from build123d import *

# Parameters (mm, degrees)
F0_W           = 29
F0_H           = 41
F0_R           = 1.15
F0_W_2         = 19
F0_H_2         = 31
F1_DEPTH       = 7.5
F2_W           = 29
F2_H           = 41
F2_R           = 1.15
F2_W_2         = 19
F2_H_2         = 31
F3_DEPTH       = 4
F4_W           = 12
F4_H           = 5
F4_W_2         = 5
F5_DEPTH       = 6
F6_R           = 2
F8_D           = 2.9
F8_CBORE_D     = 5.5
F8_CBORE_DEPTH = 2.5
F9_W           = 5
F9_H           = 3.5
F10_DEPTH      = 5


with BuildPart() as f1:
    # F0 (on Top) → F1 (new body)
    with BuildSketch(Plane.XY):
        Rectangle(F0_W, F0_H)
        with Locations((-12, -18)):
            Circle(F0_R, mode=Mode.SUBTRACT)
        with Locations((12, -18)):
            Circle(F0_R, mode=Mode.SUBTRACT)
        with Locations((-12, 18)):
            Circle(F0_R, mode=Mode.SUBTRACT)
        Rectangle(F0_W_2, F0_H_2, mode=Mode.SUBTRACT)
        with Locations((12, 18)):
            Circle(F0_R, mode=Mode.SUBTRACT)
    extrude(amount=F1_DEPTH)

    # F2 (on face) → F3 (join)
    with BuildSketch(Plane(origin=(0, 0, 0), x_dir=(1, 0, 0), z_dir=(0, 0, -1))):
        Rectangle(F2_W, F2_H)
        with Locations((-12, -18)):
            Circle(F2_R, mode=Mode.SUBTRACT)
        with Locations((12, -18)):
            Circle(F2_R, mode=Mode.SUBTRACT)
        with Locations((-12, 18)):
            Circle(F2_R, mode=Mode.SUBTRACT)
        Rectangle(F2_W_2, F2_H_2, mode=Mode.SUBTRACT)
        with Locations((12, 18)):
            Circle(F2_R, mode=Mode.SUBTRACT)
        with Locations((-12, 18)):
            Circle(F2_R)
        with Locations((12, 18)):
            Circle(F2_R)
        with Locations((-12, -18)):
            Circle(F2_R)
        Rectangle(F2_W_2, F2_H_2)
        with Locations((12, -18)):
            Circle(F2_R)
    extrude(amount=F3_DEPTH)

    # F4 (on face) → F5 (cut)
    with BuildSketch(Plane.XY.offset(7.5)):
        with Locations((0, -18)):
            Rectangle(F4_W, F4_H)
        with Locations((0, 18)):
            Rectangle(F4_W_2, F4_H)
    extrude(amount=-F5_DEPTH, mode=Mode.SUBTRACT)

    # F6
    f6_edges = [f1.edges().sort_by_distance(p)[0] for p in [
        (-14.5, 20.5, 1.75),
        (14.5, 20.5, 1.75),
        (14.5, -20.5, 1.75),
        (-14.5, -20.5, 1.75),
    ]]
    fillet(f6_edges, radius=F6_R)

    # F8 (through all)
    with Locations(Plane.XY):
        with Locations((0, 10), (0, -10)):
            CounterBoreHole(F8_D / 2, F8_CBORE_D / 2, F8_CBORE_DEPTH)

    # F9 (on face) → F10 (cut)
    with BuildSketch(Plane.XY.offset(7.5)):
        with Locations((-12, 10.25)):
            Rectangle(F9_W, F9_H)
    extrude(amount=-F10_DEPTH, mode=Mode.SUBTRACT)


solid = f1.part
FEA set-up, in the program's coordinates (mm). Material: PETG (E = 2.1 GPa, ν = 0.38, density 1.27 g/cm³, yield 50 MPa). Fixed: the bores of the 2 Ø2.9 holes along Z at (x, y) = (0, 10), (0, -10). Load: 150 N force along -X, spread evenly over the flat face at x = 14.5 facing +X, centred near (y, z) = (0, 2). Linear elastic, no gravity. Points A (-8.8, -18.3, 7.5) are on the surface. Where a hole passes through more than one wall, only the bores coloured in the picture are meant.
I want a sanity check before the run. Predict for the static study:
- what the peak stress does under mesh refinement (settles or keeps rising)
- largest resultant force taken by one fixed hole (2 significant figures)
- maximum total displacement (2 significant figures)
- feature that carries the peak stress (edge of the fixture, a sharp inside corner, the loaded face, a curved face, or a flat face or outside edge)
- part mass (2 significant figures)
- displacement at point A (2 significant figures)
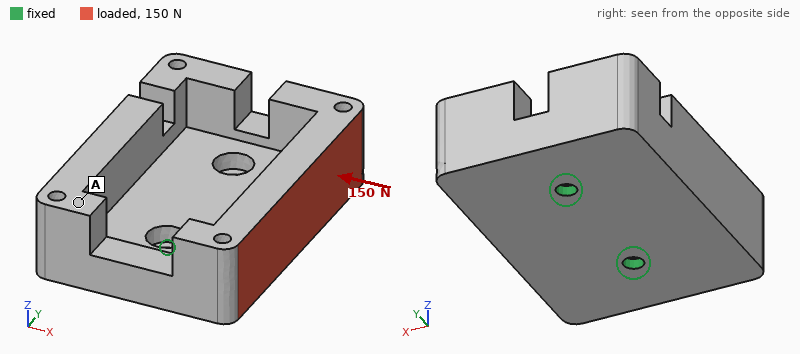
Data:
keeps rising
76 N
0.61 mm
edge of the fixture
11 g
0.38 mm
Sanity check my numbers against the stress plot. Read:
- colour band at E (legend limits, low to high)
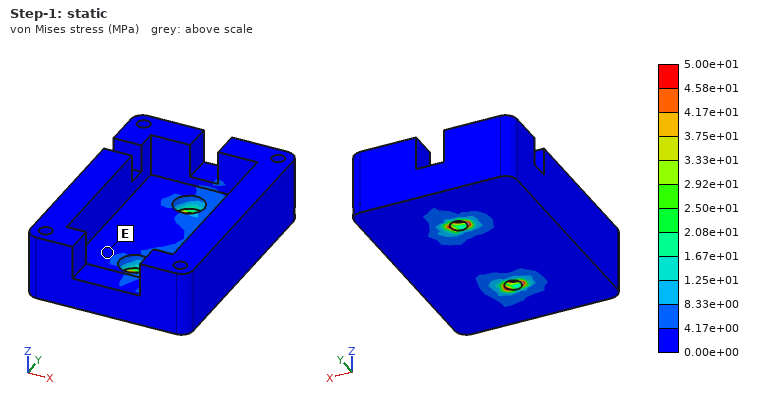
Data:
0.00e+00 to 4.17e+00 MPa
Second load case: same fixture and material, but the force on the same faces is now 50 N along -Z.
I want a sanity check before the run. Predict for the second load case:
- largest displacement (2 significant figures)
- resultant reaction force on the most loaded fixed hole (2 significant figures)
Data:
0.55 mm
25 N
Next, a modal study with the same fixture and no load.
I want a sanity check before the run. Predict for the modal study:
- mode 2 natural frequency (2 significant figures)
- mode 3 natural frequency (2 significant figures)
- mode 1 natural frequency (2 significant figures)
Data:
2200 Hz
2200 Hz
740 Hz
